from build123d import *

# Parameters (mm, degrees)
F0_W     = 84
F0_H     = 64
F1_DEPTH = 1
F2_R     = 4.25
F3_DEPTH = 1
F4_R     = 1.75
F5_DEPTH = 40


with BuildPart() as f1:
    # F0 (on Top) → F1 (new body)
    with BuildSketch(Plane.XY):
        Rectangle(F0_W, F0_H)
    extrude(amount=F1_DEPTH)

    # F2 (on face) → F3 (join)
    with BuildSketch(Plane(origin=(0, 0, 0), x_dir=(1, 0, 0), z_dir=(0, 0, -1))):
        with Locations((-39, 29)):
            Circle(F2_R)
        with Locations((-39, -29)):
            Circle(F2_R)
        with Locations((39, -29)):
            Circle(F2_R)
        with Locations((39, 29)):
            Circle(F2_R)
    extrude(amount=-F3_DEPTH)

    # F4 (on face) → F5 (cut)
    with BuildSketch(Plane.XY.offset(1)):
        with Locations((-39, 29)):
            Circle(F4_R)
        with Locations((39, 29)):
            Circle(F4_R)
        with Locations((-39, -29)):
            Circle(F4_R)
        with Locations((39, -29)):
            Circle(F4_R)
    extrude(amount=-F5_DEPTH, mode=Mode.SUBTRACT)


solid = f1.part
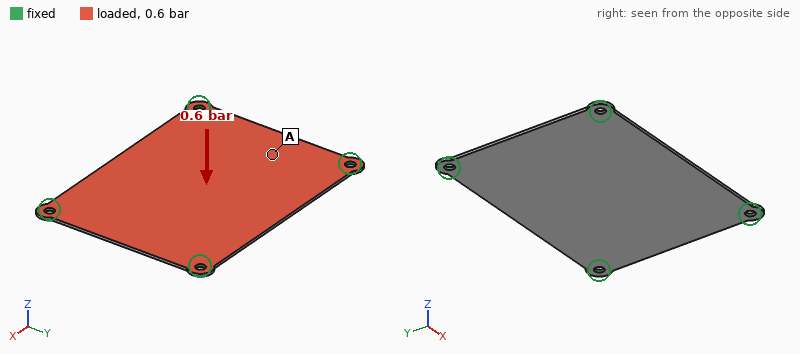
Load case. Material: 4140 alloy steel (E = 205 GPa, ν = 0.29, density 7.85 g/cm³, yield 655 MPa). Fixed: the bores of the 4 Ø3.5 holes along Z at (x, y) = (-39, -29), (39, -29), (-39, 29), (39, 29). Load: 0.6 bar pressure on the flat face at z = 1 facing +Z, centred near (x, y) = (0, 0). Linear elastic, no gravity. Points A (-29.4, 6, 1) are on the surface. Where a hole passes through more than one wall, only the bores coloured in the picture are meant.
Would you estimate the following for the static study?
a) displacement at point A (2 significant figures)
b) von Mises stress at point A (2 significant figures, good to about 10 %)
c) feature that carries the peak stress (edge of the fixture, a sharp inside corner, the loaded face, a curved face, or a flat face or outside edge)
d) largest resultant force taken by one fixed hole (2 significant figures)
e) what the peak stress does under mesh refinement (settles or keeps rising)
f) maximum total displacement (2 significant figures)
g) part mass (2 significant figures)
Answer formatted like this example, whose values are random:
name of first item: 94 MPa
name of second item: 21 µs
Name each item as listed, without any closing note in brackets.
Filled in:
displacement at point A: 0.28 mm
von Mises stress at point A: 67 MPa
feature that carries the peak stress: edge of the fixture
largest resultant force taken by one fixed hole: 81 N
what the peak stress does under mesh refinement: keeps rising
maximum total displacement: 0.60 mm
part mass: 42 g
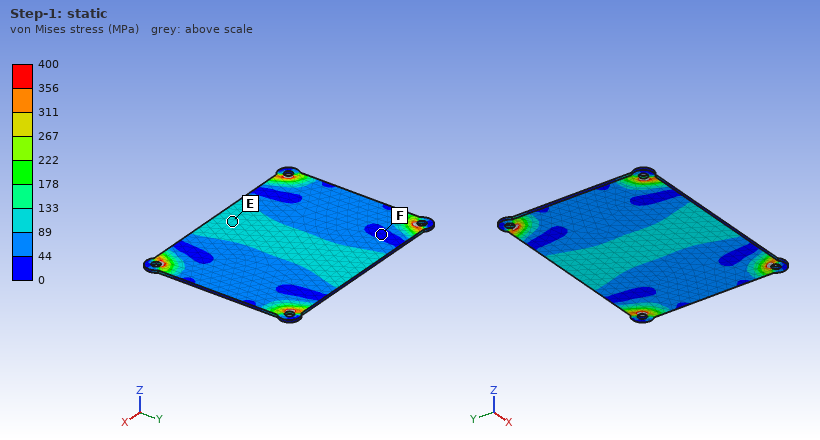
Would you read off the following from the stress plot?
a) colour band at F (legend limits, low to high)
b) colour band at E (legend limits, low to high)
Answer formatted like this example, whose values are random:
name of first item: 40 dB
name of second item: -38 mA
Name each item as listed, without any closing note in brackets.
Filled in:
colour band at F: 0 to 44 MPa
colour band at E: 89 to 133 MPa
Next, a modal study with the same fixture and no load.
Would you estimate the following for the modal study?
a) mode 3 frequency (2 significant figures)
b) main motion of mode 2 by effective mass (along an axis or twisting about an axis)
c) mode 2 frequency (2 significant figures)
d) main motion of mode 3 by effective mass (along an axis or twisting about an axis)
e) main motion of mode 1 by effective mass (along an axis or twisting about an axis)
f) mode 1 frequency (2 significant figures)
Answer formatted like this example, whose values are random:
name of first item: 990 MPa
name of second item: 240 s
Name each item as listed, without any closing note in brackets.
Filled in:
mode 3 frequency: 1500 Hz
main motion of mode 2 by effective mass: twisting about X
mode 2 frequency: 1100 Hz
main motion of mode 3 by effective mass: twisting about Y
main motion of mode 1 by effective mass: along Z
mode 1 frequency: 670 Hz
